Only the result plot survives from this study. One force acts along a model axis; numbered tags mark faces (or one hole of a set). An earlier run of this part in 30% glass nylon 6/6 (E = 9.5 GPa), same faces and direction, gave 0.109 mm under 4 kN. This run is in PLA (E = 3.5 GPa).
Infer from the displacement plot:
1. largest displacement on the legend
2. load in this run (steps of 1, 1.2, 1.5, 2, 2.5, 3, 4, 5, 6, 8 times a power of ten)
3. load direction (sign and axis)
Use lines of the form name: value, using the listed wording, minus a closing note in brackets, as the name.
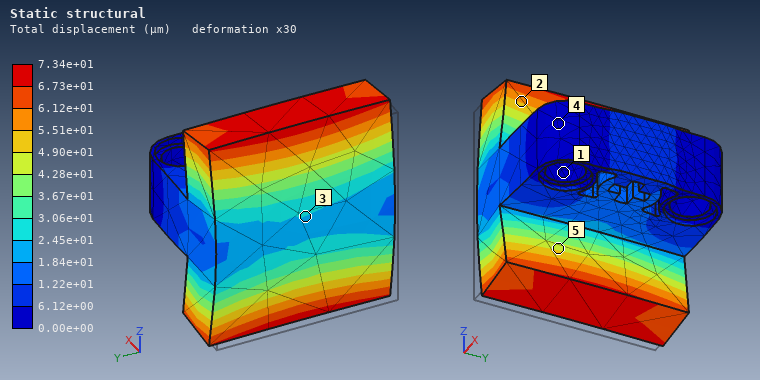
largest displacement on the legend: 7.34e+01 µm
load in this run: 1 kN
load direction: +X
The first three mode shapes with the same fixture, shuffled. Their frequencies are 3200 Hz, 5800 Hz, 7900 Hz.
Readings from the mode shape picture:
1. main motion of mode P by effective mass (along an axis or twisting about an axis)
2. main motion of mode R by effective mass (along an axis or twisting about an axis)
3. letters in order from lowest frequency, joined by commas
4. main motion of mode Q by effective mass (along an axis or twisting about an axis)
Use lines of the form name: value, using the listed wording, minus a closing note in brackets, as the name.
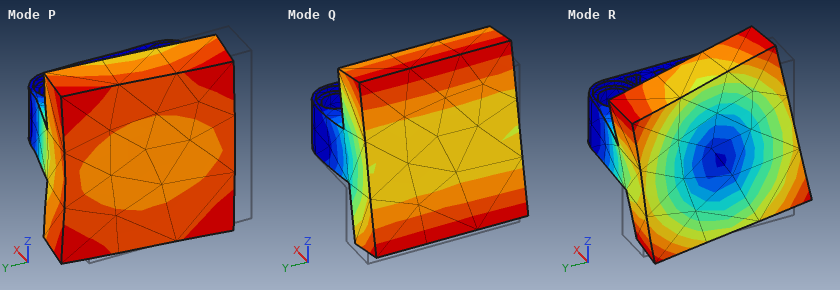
main motion of mode P by effective mass: along Y
main motion of mode R by effective mass: twisting about X
letters in order from lowest frequency, joined by commas: Q, R, P
main motion of mode Q by effective mass: along Z
